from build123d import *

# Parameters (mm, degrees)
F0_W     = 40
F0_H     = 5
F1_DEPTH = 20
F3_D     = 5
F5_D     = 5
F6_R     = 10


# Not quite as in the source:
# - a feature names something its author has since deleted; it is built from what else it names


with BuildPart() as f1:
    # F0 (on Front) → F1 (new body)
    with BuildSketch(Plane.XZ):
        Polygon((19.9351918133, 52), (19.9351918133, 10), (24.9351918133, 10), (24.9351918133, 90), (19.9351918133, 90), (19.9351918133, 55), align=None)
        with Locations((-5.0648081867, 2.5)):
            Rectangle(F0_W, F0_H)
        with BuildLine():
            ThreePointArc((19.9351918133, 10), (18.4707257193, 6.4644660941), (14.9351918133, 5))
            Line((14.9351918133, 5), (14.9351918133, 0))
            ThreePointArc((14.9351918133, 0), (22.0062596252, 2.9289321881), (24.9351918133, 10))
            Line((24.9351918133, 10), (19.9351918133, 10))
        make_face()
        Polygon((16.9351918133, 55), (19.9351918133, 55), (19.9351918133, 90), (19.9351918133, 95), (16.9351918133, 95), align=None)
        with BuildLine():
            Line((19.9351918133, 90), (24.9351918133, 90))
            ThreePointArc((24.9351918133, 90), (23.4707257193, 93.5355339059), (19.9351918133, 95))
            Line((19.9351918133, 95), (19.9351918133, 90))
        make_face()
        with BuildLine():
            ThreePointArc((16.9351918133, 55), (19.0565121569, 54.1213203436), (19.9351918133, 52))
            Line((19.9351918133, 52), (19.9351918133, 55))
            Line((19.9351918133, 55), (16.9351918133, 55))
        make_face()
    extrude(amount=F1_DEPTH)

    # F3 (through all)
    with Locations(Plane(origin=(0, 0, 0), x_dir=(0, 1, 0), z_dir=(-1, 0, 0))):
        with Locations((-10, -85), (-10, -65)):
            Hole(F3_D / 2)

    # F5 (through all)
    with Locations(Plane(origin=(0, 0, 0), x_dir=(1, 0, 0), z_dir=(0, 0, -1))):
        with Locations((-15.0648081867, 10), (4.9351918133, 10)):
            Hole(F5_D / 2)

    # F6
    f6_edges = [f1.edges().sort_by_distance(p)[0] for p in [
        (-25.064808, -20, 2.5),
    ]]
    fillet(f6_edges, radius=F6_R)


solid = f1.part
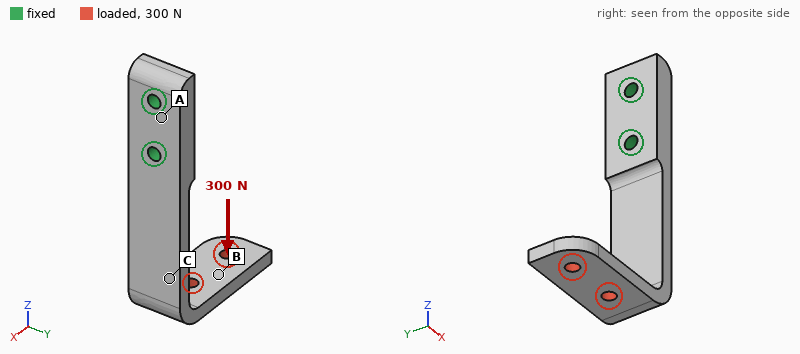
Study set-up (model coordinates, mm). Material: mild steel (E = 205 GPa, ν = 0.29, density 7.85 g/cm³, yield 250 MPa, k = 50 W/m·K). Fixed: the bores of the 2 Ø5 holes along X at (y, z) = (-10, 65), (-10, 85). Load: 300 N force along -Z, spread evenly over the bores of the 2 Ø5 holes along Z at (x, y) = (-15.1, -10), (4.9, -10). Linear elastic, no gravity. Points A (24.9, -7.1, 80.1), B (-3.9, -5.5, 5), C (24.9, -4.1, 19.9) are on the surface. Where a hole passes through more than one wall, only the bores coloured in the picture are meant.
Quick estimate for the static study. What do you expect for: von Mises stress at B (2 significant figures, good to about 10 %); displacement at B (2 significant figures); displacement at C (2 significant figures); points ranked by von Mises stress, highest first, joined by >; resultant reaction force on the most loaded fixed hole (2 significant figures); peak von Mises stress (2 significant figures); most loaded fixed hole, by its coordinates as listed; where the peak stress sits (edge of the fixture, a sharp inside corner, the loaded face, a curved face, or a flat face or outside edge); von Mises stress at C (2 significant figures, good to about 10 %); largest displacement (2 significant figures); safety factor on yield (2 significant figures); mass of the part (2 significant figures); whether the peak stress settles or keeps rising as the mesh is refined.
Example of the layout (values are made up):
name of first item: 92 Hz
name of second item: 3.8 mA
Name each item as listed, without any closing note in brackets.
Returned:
von Mises stress at B: 21 MPa
displacement at B: 0.40 mm
displacement at C: 0.14 mm
points ranked by von Mises stress, highest first, joined by >: C > B > A
resultant reaction force on the most loaded fixed hole: 270 N
peak von Mises stress: 120 MPa
most loaded fixed hole, by its coordinates as listed: (-10, 65)
where the peak stress sits: a curved face
von Mises stress at C: 95 MPa
largest displacement: 0.66 mm
safety factor on yield: 2.0
mass of the part: 120 g
whether the peak stress settles or keeps rising as the mesh is refined: settles
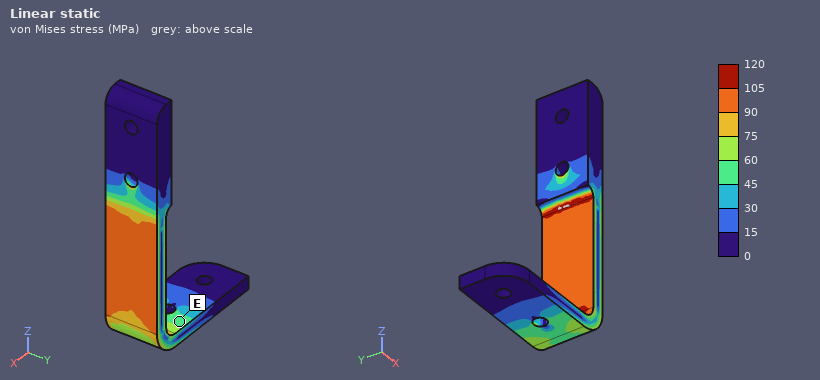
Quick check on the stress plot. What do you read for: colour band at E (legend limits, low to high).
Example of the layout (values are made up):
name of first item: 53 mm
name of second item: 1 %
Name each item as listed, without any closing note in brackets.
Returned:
colour band at E: 45 to 60 MPa
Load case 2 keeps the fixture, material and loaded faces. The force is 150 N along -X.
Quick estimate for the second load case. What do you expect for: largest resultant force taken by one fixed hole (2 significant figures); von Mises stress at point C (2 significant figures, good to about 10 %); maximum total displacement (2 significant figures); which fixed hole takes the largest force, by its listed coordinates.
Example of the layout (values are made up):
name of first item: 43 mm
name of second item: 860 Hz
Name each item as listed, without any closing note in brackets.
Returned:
largest resultant force taken by one fixed hole: 260 N
von Mises stress at point C: 31 MPa
maximum total displacement: 0.33 mm
which fixed hole takes the largest force, by its listed coordinates: (-10, 65)
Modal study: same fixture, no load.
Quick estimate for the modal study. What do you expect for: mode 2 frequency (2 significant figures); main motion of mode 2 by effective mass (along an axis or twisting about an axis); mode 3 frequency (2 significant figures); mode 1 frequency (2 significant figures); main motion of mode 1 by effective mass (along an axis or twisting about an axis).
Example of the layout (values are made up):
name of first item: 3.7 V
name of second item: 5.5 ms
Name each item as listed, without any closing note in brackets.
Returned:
mode 2 frequency: 950 Hz
main motion of mode 2 by effective mass: along Y
mode 3 frequency: 1600 Hz
mode 1 frequency: 550 Hz
main motion of mode 1 by effective mass: along X
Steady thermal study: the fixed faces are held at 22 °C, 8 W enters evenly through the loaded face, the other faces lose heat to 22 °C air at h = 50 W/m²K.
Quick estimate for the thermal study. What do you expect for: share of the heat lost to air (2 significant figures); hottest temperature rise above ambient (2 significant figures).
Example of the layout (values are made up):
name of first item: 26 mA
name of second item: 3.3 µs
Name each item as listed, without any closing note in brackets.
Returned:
share of the heat lost to air: 78 %
hottest temperature rise above ambient: 49 K
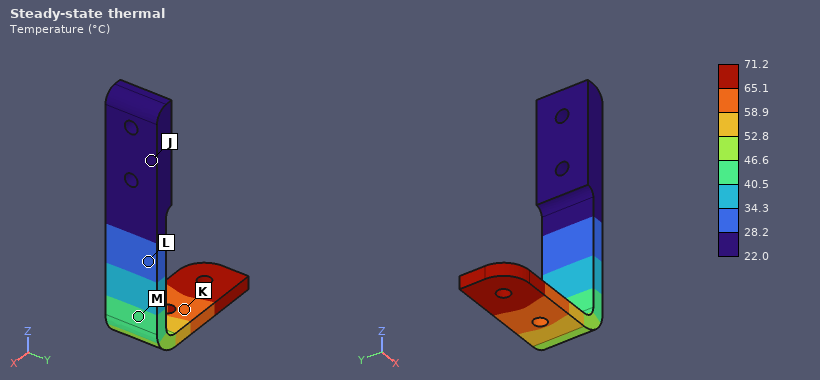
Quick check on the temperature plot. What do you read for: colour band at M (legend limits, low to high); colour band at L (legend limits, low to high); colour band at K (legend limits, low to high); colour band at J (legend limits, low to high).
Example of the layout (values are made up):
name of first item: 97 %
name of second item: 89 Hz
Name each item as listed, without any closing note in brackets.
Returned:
colour band at M: 40.5 to 46.6 °C
colour band at L: 28.2 to 34.3 °C
colour band at K: 58.9 to 65.1 °C
colour band at J: 22.0 to 28.2 °C
